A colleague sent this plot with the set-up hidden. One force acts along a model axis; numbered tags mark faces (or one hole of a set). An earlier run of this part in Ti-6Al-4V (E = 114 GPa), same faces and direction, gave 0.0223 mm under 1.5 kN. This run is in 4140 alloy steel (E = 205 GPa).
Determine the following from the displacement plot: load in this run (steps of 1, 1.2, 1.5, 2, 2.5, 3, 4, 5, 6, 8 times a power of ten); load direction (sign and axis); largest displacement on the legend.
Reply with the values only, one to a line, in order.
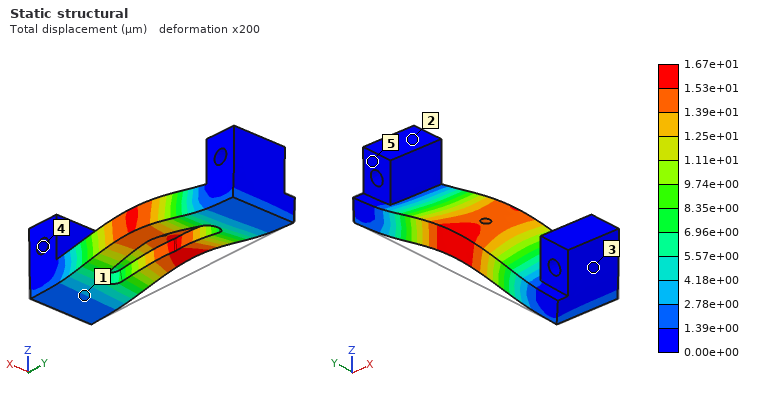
2 kN
+Z
1.67e+01 µm
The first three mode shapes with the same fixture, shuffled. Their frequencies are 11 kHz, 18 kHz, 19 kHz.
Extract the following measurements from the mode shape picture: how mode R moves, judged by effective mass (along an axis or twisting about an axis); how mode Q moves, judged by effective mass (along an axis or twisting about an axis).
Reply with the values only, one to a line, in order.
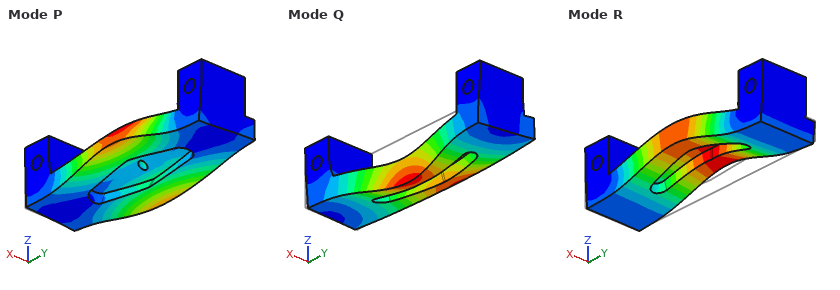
along Z
along X
